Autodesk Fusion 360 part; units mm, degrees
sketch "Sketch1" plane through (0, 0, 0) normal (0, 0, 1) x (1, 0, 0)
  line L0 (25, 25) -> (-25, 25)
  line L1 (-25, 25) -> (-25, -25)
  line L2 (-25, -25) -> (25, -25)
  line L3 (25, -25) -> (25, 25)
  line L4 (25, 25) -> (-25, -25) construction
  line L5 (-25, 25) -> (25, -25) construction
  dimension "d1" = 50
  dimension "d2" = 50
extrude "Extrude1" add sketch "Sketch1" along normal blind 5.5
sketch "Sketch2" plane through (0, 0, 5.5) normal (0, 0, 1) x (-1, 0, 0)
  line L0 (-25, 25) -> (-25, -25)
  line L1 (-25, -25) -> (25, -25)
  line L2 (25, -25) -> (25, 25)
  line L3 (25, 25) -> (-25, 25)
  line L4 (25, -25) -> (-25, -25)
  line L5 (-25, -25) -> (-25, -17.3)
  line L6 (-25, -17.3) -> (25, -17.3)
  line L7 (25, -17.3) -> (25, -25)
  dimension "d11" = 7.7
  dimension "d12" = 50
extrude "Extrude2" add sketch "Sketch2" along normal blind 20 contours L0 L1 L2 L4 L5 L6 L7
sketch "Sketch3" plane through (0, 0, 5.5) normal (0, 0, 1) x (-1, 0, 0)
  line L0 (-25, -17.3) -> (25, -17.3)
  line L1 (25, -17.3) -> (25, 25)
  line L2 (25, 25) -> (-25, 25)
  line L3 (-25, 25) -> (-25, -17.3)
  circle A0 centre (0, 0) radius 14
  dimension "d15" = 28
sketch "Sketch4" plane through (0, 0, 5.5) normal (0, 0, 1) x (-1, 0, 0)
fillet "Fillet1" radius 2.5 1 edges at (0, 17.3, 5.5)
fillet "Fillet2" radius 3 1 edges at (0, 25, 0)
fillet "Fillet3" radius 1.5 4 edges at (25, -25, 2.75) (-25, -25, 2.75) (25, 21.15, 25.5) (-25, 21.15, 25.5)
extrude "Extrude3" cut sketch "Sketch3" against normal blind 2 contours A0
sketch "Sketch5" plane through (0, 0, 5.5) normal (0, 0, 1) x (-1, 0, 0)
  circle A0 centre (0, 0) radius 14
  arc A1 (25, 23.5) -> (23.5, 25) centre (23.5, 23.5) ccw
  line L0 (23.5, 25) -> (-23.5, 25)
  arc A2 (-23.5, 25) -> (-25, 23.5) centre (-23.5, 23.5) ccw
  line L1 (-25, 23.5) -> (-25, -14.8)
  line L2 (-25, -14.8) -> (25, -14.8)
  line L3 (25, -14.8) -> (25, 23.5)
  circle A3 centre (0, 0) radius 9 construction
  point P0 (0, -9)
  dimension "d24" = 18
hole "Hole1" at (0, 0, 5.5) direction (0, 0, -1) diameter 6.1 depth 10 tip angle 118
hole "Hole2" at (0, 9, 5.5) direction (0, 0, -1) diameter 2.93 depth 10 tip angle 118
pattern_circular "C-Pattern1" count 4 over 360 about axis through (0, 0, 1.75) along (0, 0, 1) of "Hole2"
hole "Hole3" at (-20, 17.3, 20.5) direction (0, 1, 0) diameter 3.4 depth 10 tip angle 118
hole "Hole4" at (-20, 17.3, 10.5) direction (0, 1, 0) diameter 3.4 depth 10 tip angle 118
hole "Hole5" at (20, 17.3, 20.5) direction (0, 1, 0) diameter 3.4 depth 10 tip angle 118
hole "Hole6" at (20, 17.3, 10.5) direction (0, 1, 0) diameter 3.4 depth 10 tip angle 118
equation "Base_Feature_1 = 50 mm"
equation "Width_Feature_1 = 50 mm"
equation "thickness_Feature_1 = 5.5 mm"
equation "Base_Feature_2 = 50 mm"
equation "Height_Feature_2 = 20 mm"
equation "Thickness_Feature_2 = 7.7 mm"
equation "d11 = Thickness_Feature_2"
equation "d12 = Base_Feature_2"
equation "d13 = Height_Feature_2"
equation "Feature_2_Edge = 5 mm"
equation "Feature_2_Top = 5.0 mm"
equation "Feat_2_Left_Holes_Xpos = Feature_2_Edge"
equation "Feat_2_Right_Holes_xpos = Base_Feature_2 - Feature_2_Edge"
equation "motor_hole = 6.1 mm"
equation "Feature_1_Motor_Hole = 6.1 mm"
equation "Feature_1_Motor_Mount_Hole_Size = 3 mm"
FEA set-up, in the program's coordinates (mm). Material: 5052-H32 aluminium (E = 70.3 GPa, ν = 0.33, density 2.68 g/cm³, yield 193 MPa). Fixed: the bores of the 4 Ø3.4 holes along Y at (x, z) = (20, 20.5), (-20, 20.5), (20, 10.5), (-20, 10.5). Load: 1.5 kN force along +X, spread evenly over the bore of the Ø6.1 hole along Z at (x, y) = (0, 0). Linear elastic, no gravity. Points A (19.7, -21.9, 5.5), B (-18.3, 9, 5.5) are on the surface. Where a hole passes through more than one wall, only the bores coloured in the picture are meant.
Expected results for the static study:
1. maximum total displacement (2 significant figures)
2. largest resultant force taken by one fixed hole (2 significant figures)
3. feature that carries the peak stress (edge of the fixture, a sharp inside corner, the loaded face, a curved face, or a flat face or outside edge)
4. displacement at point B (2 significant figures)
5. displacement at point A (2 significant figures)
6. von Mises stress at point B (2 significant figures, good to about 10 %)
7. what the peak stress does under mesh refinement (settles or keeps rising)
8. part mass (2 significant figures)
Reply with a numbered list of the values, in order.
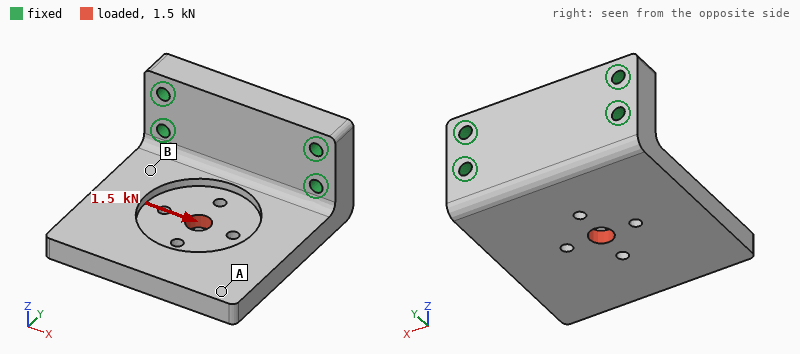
1. 24 µm
2. 1.0 kN
3. edge of the fixture
4. 8.8 µm
5. 22 µm
6. 12 MPa
7. keeps rising
8. 53 g
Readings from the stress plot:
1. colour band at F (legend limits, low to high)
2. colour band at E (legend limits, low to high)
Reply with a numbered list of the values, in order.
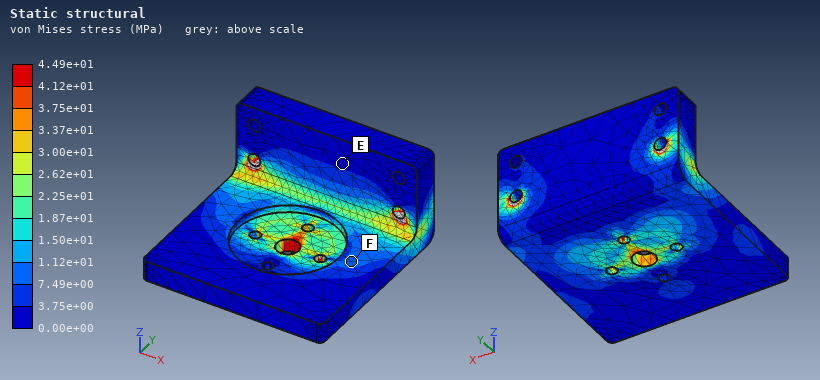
1. 7.49e+00 to 1.12e+01 MPa
2. 0.00e+00 to 3.75e+00 MPa
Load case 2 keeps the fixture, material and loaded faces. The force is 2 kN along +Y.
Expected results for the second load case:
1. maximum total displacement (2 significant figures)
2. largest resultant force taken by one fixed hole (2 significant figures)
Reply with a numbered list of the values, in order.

1. 72 µm
2. 1.2 kN
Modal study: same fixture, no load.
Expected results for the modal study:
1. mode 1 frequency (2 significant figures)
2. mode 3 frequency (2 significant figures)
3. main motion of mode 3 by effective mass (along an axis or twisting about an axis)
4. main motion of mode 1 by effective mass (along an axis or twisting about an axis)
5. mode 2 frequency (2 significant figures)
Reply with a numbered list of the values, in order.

1. 1900 Hz
2. 8300 Hz
3. along X
4. along Z
5. 4200 Hz
